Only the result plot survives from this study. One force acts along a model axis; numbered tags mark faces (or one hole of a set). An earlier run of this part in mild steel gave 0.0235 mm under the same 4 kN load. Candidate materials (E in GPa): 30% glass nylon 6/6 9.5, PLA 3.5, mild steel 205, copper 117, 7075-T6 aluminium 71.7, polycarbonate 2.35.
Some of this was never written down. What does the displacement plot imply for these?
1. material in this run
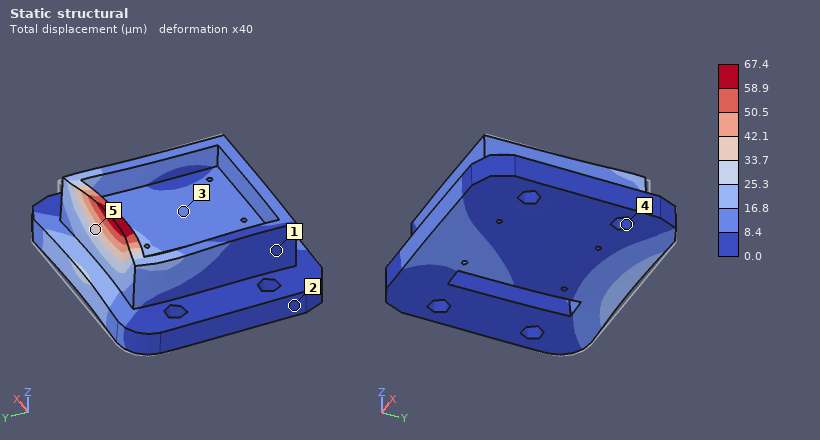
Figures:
7075-T6 aluminium
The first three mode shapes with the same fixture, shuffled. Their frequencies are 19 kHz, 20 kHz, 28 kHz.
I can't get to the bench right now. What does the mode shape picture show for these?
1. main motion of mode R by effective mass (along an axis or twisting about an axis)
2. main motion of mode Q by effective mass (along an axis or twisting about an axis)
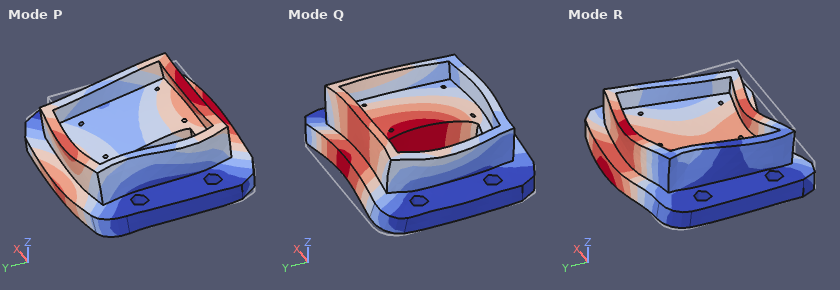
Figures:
along Y
along Z
